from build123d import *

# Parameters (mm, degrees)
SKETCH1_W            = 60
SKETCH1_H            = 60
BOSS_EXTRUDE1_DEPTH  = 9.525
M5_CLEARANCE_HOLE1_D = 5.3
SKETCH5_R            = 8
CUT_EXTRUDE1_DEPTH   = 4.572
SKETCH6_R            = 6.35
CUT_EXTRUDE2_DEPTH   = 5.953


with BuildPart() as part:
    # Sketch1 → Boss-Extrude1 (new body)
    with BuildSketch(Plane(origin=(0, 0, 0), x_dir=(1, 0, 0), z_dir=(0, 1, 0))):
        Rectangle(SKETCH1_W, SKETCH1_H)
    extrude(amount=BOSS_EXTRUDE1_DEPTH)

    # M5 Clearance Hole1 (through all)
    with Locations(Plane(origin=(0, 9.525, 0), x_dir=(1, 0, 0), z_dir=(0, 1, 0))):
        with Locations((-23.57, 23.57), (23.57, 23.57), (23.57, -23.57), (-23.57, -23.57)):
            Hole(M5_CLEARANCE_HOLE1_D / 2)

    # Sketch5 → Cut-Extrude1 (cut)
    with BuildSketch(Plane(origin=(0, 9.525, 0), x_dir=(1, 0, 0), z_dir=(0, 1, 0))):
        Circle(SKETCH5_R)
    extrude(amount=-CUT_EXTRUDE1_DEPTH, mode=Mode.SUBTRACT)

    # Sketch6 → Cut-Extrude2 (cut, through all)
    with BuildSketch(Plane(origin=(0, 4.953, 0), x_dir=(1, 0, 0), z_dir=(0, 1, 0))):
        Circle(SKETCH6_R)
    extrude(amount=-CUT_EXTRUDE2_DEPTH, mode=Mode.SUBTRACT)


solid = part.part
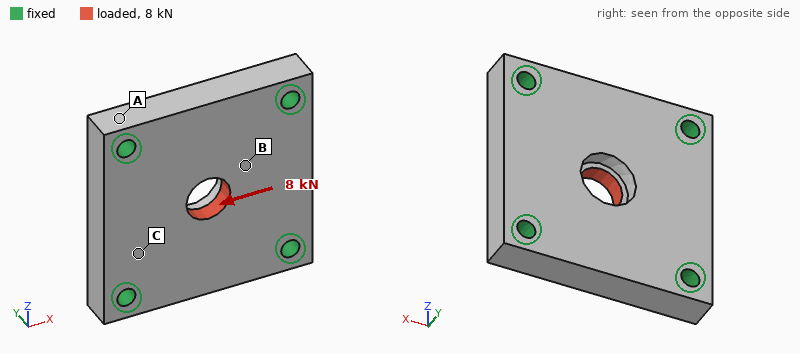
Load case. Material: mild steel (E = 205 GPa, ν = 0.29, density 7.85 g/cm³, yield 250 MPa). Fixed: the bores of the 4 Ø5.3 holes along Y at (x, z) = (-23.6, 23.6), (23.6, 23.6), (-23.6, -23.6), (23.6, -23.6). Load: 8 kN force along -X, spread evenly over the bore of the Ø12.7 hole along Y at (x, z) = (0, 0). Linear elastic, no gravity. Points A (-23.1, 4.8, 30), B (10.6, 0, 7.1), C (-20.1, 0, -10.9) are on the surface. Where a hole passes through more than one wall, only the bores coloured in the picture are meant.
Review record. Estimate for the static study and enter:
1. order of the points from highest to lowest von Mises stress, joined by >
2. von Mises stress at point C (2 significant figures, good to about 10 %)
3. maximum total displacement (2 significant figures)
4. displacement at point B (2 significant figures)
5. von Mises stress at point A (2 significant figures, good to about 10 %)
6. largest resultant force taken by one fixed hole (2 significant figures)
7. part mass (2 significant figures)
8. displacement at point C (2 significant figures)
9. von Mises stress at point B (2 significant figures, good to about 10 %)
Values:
B > C > A
15 MPa
3.9 µm
2.3 µm
7.4 MPa
2.2 kN
250 g
1.6 µm
27 MPa
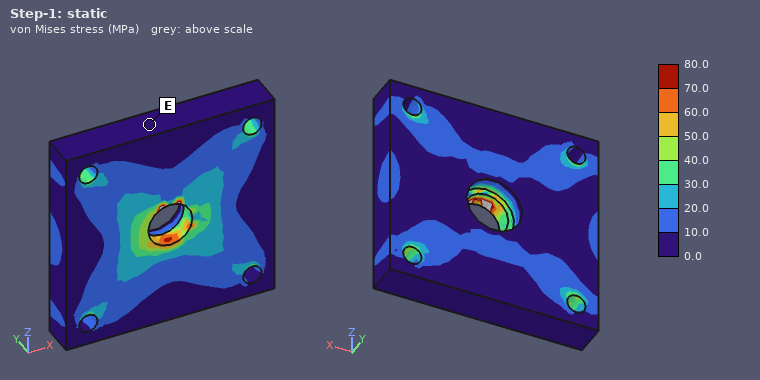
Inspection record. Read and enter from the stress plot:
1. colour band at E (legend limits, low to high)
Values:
0.0 to 10.0 MPa
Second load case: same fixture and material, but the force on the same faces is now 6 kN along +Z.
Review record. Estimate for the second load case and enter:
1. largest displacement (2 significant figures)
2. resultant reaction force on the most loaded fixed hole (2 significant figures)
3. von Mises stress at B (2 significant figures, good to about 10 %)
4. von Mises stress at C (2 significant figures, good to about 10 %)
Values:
2.9 µm
1.7 kN
17 MPa
10 MPa
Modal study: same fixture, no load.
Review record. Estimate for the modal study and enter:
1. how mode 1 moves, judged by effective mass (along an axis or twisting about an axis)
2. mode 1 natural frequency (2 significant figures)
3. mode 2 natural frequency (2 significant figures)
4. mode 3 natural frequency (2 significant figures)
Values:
along Y
13 kHz
20 kHz
20 kHz
